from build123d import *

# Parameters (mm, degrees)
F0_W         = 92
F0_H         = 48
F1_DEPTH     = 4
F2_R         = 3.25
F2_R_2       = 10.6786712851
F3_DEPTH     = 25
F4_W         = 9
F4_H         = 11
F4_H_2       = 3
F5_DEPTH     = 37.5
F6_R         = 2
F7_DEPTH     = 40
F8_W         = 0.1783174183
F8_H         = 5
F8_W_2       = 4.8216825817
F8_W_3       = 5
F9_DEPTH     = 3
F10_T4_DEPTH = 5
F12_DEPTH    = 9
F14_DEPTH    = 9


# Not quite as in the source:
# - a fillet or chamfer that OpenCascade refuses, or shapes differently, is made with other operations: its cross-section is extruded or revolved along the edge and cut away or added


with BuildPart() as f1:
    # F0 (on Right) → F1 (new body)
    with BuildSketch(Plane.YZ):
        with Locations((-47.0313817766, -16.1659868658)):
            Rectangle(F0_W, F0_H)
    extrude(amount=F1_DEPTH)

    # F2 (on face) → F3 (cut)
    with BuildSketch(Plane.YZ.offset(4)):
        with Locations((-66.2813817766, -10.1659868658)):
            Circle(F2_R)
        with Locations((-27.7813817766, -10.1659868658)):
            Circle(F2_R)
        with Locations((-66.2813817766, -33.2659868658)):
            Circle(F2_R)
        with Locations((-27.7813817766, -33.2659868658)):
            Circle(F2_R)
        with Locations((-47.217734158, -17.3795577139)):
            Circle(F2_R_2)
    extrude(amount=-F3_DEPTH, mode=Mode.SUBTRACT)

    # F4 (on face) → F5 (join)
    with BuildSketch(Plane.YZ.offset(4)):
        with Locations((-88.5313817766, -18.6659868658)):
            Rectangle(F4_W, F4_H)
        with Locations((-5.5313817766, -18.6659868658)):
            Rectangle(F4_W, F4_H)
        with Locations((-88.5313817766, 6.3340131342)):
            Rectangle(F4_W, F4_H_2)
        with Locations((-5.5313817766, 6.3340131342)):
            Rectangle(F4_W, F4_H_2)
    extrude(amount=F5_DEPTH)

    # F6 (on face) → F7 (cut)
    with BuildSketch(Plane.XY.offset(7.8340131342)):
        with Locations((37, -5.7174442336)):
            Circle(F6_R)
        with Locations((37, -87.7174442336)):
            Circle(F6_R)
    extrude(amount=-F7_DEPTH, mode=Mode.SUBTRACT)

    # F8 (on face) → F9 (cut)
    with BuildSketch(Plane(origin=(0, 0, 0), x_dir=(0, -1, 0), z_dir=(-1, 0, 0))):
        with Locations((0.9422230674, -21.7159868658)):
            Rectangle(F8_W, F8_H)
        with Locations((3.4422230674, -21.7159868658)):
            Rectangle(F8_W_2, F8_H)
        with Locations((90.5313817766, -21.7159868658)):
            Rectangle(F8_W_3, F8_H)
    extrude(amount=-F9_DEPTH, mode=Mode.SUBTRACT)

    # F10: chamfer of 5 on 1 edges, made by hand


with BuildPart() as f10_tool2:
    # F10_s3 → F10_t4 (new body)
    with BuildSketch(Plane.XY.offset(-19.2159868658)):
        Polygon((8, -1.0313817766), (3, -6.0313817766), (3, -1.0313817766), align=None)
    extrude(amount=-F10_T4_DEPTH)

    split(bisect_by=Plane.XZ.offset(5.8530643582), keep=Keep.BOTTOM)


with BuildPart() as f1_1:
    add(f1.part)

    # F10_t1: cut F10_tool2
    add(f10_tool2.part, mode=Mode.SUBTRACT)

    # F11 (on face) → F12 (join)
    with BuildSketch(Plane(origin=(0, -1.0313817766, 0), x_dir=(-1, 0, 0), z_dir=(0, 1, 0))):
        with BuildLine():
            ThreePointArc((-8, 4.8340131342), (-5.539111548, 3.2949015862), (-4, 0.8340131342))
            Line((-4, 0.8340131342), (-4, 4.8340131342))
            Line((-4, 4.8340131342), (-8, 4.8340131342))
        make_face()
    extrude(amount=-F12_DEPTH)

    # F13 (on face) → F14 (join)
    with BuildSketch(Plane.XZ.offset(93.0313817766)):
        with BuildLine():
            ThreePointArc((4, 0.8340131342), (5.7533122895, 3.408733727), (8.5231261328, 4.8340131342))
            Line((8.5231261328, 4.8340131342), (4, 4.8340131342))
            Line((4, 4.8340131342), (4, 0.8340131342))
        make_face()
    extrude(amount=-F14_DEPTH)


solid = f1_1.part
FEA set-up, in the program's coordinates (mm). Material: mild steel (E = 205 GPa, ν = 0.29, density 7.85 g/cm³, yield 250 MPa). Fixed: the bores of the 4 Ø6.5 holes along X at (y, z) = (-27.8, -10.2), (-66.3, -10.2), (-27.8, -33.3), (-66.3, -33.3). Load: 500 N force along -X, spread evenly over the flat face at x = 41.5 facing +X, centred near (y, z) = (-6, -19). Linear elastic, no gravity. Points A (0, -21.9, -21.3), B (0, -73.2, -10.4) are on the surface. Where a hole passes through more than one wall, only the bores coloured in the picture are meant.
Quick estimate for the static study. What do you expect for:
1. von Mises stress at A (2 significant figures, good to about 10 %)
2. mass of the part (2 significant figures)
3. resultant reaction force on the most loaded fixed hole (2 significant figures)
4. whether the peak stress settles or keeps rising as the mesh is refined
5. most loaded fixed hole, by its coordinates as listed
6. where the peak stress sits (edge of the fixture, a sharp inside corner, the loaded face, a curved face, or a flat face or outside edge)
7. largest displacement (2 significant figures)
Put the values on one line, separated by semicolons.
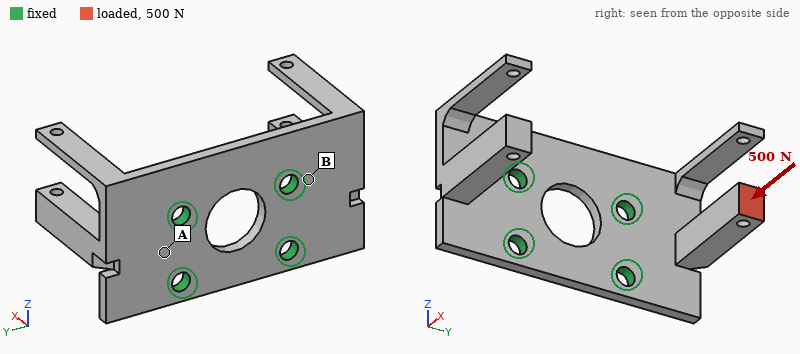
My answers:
53 MPa; 190 g; 330 N; keeps rising; (-27.8, -10.2); a sharp inside corner; 0.10 mm
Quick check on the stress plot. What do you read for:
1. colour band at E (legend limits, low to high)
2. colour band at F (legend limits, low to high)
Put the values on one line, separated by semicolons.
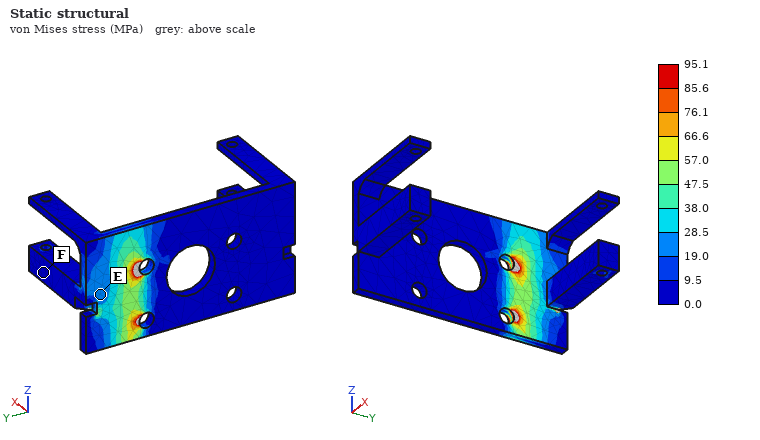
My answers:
19.0 to 28.5 MPa; 0.0 to 9.5 MPa
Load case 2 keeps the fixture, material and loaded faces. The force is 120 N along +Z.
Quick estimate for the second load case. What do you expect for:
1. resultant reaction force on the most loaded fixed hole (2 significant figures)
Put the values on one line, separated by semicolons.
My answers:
220 N
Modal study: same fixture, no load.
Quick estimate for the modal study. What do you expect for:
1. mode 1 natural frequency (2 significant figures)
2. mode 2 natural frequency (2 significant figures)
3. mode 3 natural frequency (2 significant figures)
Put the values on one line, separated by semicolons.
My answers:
1500 Hz; 1500 Hz; 1700 Hz
